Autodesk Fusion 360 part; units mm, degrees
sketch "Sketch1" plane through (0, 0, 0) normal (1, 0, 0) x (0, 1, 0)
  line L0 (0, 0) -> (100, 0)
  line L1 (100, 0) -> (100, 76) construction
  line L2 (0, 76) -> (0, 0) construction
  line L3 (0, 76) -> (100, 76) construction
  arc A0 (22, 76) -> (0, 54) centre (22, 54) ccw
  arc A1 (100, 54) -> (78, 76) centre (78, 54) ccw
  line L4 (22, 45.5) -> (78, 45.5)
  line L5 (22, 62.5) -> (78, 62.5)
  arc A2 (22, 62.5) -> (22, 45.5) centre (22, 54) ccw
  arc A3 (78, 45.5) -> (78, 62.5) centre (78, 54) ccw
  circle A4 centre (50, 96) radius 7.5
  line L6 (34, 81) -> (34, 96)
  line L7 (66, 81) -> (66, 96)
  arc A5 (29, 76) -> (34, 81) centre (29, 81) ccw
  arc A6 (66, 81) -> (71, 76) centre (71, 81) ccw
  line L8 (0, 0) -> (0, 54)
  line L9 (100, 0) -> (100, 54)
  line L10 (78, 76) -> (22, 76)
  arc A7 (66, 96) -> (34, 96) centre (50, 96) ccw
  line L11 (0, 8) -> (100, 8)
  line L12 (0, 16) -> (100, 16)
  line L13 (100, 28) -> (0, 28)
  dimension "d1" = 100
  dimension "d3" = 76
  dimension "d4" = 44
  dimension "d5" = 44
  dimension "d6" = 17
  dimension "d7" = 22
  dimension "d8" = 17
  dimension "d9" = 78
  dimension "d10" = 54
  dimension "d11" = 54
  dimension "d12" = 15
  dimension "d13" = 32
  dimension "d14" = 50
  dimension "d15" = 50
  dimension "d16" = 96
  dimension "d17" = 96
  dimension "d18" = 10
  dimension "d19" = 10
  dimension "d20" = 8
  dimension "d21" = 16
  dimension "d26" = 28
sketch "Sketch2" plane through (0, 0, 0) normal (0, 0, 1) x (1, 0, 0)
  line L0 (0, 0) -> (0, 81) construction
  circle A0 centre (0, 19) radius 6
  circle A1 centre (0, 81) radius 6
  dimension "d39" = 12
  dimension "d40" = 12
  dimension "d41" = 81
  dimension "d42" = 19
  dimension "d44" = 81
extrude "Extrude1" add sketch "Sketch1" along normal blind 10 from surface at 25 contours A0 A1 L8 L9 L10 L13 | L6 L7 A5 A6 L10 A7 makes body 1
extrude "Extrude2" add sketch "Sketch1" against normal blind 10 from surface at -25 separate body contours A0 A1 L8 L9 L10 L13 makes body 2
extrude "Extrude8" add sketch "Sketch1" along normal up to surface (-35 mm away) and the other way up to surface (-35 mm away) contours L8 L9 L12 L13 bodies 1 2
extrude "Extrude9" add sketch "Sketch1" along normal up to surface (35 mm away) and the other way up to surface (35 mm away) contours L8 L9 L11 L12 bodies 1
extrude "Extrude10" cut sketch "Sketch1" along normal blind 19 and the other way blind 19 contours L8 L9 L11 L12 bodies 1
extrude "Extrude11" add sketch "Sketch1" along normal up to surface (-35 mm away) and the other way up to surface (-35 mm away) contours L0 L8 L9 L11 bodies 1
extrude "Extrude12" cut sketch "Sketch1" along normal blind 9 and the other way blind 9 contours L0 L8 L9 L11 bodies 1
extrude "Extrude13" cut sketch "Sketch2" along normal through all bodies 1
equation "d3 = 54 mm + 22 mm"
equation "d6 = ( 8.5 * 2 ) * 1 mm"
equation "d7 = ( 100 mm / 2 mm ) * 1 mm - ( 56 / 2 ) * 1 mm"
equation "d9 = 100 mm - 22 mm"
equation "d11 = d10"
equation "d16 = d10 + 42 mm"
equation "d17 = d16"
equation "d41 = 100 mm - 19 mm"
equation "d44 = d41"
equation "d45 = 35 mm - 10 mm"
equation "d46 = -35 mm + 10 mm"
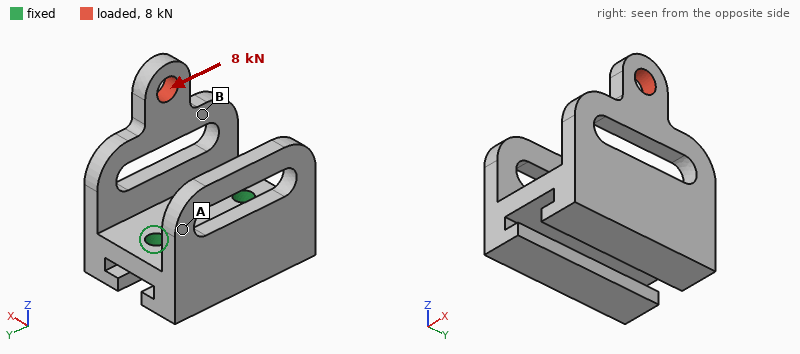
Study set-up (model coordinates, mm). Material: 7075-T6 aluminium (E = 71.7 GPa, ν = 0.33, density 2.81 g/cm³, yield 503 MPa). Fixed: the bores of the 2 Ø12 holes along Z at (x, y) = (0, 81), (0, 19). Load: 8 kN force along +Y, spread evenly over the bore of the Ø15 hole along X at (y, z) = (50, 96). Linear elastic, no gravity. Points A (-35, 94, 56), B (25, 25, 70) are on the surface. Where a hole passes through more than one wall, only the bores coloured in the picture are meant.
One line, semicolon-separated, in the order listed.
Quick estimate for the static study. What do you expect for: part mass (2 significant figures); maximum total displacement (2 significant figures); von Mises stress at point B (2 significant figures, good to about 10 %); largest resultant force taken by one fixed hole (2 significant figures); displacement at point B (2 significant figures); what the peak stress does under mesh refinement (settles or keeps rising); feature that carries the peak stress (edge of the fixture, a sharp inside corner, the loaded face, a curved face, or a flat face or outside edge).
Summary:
630 g; 0.47 mm; 100 MPa; 9.7 kN; 0.23 mm; keeps rising; edge of the fixture
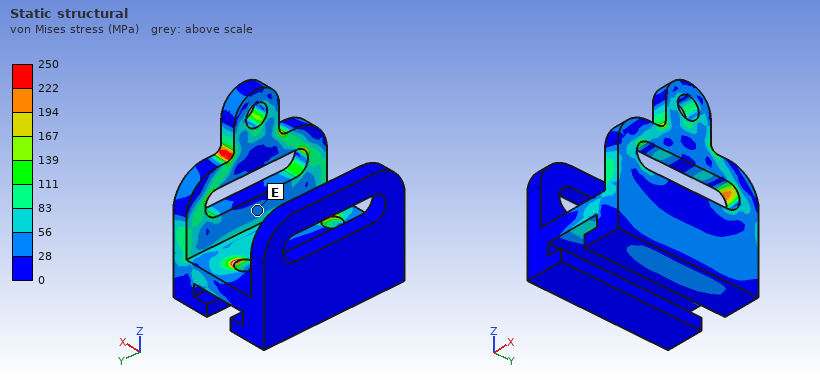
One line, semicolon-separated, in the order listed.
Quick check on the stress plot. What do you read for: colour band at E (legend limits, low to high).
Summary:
28 to 56 MPa
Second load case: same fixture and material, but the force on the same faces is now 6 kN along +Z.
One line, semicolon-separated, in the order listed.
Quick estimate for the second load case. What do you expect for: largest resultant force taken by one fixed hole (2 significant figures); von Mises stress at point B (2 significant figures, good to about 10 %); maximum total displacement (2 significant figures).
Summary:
3.0 kN; 63 MPa; 0.28 mm
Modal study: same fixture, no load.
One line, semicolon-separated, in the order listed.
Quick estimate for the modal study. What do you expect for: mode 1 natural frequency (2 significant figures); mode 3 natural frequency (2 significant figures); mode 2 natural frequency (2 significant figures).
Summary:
1000 Hz; 3000 Hz; 1800 Hz
